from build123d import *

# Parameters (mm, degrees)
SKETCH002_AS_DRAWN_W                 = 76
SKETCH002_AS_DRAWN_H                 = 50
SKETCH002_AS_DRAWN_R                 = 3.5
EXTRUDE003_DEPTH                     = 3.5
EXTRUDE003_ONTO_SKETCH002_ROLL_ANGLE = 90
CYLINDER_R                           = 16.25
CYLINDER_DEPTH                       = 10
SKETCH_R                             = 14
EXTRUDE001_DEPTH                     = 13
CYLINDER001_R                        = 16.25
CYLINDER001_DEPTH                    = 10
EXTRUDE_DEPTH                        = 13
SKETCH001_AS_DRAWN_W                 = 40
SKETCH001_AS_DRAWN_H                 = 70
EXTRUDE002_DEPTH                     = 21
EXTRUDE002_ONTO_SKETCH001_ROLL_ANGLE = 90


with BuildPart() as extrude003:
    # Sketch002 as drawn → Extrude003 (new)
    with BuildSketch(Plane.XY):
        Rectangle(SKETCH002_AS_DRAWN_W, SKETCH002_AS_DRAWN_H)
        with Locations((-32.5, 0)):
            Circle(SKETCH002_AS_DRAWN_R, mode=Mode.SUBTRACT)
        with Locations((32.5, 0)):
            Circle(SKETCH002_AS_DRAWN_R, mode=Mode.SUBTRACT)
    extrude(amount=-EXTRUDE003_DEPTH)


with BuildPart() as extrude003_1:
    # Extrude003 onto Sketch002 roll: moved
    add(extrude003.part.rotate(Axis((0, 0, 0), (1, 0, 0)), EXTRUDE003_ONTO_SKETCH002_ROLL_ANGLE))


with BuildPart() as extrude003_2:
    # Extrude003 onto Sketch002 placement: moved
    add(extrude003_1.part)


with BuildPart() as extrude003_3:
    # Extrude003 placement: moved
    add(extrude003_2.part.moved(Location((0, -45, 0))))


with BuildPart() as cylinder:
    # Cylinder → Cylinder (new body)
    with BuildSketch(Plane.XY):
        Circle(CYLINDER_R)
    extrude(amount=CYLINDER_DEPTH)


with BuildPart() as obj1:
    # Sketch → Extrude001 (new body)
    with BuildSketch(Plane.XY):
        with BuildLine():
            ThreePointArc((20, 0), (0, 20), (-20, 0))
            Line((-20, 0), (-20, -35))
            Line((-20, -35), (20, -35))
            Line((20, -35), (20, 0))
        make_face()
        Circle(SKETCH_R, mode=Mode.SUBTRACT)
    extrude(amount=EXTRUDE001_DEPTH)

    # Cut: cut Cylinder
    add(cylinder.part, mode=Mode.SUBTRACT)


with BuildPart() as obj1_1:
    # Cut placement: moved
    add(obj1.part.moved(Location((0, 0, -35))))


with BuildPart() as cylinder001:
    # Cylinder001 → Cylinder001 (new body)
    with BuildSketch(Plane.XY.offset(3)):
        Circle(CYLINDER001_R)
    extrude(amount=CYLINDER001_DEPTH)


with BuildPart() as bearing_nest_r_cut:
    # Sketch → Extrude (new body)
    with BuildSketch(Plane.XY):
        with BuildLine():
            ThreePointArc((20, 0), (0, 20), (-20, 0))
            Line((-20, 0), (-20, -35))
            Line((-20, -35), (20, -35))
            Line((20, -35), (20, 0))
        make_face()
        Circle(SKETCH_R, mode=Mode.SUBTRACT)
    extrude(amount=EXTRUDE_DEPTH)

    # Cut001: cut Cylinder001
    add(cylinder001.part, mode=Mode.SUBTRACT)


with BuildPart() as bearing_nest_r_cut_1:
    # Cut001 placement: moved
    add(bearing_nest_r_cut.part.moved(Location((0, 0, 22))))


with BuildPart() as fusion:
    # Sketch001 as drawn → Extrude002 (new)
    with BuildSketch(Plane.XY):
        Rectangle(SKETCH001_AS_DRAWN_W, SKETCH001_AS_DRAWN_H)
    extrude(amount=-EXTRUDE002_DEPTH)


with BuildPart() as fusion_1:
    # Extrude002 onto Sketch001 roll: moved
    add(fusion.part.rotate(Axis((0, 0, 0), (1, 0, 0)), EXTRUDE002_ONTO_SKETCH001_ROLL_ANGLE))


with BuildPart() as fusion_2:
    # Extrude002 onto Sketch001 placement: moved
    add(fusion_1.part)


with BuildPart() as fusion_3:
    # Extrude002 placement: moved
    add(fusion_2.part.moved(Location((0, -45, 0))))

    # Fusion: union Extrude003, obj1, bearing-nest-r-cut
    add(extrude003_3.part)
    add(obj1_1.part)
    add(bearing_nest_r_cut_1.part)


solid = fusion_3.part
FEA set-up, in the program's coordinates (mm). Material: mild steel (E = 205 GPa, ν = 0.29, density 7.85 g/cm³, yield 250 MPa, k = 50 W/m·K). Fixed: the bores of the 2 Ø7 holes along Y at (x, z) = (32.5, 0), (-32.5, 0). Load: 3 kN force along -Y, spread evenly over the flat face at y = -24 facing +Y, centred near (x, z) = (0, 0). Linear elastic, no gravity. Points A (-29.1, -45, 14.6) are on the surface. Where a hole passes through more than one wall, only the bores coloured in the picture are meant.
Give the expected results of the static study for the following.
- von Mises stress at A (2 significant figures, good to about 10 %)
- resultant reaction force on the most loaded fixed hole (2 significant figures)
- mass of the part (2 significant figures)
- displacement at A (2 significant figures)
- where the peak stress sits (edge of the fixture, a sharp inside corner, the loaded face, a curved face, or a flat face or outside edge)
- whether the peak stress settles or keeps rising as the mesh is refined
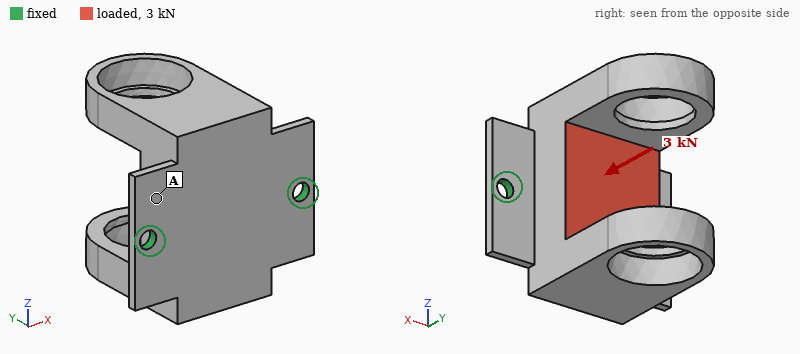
17 MPa
1.7 kN
670 g
9.1 µm
edge of the fixture
keeps rising
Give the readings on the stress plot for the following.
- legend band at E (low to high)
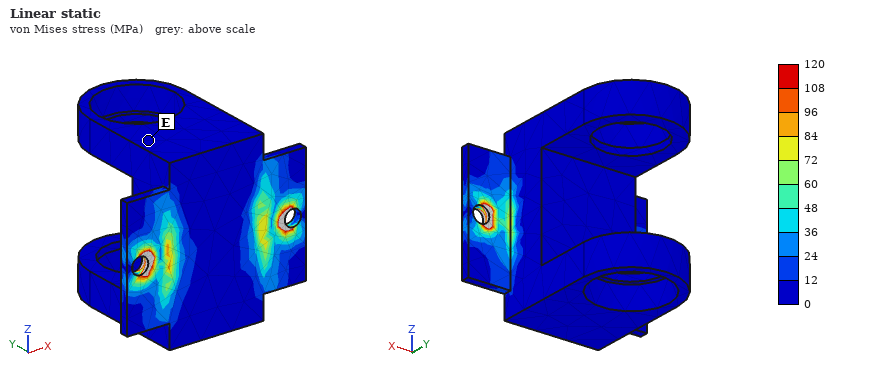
0 to 12 MPa
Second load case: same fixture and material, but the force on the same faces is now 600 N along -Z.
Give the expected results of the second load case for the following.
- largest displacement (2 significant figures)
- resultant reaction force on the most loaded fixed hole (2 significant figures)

83 µm
300 N
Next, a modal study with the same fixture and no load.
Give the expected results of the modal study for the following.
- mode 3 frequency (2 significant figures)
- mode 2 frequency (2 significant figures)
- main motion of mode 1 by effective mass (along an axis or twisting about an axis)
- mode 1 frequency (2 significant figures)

2600 Hz
2600 Hz
along Z
640 Hz
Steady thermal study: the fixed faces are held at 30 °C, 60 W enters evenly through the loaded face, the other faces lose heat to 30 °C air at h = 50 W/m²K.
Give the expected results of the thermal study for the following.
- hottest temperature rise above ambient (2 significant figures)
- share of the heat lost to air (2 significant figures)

49 K
54 %
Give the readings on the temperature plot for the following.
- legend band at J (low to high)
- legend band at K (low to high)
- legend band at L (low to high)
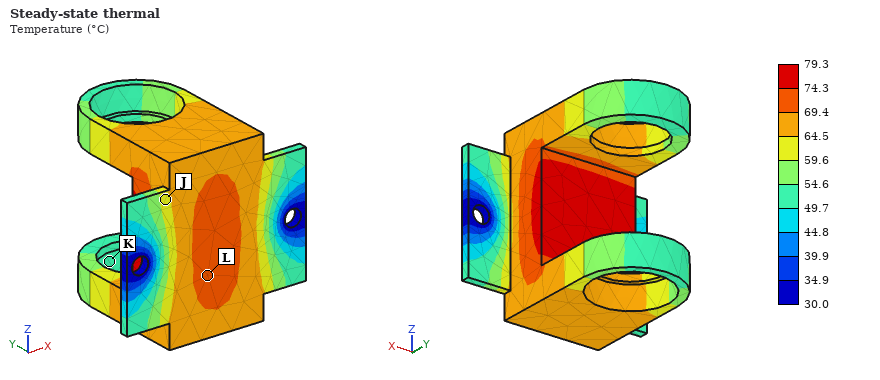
59.6 to 64.5 °C
49.7 to 54.6 °C
69.4 to 74.3 °C
